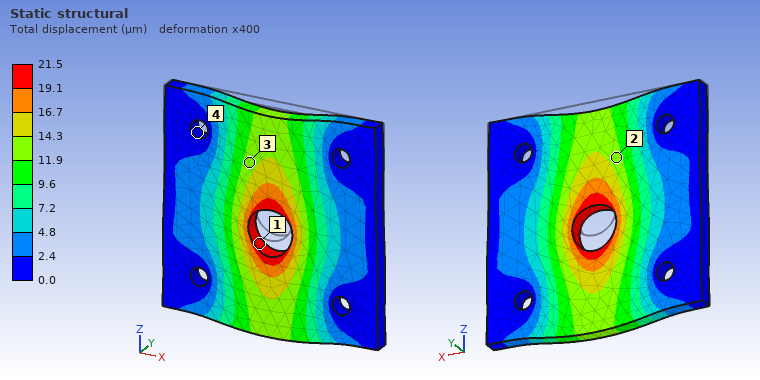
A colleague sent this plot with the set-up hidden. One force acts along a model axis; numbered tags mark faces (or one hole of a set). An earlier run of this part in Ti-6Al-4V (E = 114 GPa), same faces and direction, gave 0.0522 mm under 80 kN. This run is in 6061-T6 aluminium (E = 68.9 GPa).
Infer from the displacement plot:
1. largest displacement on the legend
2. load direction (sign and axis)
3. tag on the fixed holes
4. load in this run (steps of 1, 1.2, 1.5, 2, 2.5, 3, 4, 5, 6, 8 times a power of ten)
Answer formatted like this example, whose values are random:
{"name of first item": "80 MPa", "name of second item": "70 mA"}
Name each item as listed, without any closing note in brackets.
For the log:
{"largest displacement on the legend": "21.5 µm", "load direction": "-Z", "tag on the fixed holes": "4", "load in this run": "20 kN"}
